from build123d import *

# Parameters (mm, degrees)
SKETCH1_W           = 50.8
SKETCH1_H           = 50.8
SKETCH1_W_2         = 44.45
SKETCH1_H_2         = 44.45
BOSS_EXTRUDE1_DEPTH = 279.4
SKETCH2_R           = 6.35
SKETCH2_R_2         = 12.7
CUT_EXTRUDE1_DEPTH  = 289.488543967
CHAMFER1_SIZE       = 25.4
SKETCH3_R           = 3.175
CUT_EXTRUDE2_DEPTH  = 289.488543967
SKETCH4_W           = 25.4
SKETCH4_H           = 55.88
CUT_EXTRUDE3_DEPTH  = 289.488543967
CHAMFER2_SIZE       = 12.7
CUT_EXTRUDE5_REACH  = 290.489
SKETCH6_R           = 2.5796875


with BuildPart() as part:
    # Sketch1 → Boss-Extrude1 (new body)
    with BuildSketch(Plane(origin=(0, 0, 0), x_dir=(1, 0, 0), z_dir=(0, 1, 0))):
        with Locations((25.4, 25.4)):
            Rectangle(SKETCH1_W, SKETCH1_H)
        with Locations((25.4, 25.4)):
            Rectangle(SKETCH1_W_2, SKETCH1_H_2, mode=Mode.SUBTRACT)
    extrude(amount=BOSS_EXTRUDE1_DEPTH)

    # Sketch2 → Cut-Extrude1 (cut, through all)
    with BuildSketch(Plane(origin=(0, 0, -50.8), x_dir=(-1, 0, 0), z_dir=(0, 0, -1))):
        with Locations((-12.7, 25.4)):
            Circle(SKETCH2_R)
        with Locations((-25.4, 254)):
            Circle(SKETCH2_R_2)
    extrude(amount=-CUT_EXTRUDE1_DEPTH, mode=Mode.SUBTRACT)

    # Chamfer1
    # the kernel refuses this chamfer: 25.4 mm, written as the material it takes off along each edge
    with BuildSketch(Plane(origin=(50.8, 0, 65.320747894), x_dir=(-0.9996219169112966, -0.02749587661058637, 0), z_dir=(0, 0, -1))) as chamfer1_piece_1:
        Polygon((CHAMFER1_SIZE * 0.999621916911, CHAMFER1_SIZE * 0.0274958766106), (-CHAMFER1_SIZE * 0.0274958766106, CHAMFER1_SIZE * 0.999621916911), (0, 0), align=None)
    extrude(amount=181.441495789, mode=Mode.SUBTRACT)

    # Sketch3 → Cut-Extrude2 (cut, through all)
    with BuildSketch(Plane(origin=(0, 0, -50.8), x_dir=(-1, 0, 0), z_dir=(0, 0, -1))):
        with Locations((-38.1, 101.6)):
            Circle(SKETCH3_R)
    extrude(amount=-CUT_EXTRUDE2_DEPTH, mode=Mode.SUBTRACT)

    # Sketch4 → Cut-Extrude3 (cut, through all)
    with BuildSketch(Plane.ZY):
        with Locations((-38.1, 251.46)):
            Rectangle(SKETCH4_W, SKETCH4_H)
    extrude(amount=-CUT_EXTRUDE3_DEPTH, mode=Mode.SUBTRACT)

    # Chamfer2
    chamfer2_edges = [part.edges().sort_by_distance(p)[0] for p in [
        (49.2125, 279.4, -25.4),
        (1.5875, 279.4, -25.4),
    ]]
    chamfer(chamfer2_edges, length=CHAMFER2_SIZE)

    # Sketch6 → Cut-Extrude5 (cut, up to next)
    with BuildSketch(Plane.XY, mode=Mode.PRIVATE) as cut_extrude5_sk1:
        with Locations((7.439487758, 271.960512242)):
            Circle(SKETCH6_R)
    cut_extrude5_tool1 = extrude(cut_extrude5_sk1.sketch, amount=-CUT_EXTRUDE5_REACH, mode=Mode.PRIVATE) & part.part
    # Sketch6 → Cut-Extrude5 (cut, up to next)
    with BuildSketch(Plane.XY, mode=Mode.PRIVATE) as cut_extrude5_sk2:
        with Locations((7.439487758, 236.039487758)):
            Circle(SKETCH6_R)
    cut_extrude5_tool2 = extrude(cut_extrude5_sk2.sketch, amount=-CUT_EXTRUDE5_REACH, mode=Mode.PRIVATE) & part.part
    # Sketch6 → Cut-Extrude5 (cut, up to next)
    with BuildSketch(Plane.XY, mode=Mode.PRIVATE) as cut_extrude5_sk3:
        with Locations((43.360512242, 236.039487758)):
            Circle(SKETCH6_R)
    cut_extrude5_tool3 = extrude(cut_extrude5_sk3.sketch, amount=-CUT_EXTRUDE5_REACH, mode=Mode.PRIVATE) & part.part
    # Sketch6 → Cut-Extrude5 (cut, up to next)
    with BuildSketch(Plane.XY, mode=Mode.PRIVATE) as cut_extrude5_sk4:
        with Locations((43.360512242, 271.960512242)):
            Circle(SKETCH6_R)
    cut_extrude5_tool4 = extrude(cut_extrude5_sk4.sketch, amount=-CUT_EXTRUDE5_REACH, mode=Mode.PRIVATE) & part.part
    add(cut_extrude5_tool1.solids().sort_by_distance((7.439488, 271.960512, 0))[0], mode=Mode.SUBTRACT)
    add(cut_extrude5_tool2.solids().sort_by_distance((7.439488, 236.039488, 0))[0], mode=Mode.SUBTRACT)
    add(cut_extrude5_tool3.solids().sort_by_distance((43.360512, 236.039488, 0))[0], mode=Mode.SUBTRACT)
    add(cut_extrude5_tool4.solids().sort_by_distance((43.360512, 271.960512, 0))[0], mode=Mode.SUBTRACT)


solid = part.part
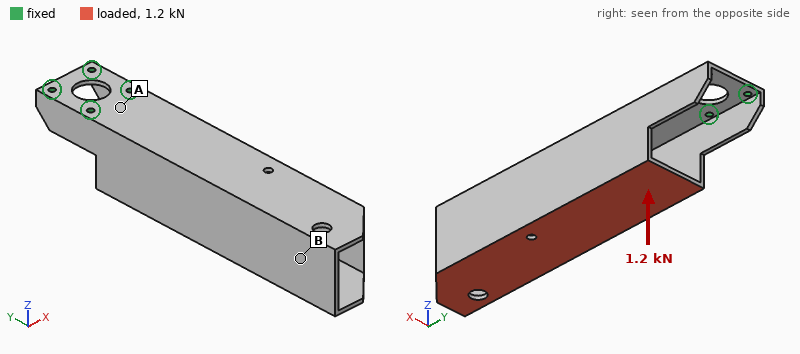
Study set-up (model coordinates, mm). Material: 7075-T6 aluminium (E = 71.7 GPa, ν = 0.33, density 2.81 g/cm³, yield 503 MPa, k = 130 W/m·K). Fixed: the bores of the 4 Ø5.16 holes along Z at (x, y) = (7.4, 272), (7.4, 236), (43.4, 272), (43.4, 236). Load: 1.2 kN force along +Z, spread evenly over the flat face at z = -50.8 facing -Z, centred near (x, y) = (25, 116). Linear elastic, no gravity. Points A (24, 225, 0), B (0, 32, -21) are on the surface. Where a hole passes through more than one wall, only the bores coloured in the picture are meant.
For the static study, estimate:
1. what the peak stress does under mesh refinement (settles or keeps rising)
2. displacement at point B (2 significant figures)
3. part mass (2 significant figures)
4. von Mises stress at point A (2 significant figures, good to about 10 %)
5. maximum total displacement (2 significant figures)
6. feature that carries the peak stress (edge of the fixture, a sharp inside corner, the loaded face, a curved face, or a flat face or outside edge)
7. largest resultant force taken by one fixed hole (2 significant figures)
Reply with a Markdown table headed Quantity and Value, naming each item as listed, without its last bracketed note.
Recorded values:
| Quantity | Value |
|---|---|
| what the peak stress does under mesh refinement | keeps rising |
| displacement at point B | 1.3 mm |
| part mass | 400 g |
| von Mises stress at point A | 45 MPa |
| maximum total displacement | 1.6 mm |
| feature that carries the peak stress | edge of the fixture |
| largest resultant force taken by one fixed hole | 2.9 kN |
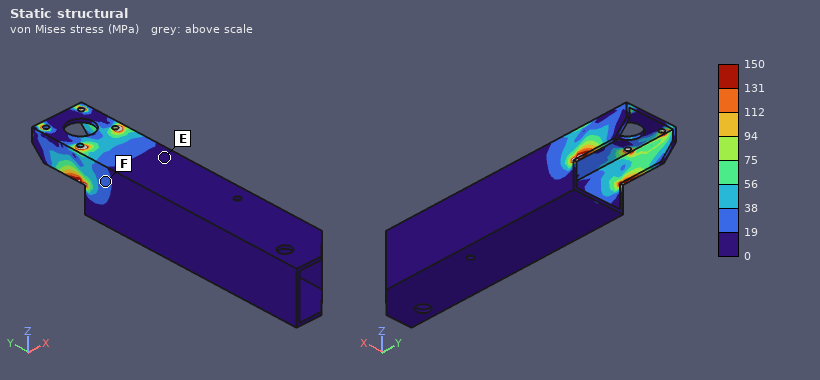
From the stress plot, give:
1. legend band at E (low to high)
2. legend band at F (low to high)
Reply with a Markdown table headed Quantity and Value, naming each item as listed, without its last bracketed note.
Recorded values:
| Quantity | Value |
|---|---|
| legend band at E | 0 to 19 MPa |
| legend band at F | 19 to 38 MPa |
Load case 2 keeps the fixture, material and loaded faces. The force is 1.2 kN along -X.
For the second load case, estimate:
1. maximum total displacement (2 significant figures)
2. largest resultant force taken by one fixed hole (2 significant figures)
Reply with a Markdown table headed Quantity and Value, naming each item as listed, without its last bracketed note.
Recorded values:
| Quantity | Value |
|---|---|
| maximum total displacement | 0.62 mm |
| largest resultant force taken by one fixed hole | 3.2 kN |
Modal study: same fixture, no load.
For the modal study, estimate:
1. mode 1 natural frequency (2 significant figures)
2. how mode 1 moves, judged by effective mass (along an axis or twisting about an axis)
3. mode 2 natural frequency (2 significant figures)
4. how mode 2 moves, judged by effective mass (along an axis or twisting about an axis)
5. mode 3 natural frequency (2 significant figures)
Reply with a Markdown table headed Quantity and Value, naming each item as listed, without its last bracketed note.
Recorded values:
| Quantity | Value |
|---|---|
| mode 1 natural frequency | 290 Hz |
| how mode 1 moves, judged by effective mass | along Z |
| mode 2 natural frequency | 540 Hz |
| how mode 2 moves, judged by effective mass | along X |
| mode 3 natural frequency | 790 Hz |
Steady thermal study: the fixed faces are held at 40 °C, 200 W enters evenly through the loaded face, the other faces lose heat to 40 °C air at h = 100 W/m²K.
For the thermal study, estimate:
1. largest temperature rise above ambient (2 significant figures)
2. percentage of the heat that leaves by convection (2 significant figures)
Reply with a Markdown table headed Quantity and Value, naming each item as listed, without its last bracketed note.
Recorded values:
| Quantity | Value |
|---|---|
| largest temperature rise above ambient | 53 K |
| percentage of the heat that leaves by convection | 94 % |
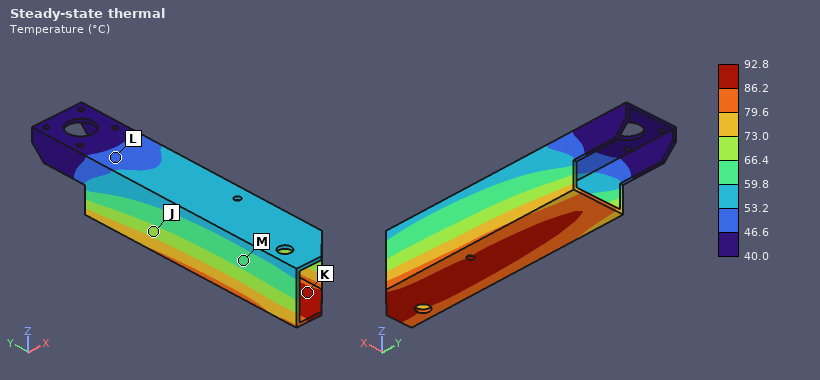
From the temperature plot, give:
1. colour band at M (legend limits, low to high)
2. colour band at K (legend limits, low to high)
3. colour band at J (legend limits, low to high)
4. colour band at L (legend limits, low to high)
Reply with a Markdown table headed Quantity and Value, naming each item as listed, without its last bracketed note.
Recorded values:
| Quantity | Value |
|---|---|
| colour band at M | 59.8 to 66.4 °C |
| colour band at K | 86.2 to 92.8 °C |
| colour band at J | 66.4 to 73.0 °C |
| colour band at L | 46.6 to 53.2 °C |
